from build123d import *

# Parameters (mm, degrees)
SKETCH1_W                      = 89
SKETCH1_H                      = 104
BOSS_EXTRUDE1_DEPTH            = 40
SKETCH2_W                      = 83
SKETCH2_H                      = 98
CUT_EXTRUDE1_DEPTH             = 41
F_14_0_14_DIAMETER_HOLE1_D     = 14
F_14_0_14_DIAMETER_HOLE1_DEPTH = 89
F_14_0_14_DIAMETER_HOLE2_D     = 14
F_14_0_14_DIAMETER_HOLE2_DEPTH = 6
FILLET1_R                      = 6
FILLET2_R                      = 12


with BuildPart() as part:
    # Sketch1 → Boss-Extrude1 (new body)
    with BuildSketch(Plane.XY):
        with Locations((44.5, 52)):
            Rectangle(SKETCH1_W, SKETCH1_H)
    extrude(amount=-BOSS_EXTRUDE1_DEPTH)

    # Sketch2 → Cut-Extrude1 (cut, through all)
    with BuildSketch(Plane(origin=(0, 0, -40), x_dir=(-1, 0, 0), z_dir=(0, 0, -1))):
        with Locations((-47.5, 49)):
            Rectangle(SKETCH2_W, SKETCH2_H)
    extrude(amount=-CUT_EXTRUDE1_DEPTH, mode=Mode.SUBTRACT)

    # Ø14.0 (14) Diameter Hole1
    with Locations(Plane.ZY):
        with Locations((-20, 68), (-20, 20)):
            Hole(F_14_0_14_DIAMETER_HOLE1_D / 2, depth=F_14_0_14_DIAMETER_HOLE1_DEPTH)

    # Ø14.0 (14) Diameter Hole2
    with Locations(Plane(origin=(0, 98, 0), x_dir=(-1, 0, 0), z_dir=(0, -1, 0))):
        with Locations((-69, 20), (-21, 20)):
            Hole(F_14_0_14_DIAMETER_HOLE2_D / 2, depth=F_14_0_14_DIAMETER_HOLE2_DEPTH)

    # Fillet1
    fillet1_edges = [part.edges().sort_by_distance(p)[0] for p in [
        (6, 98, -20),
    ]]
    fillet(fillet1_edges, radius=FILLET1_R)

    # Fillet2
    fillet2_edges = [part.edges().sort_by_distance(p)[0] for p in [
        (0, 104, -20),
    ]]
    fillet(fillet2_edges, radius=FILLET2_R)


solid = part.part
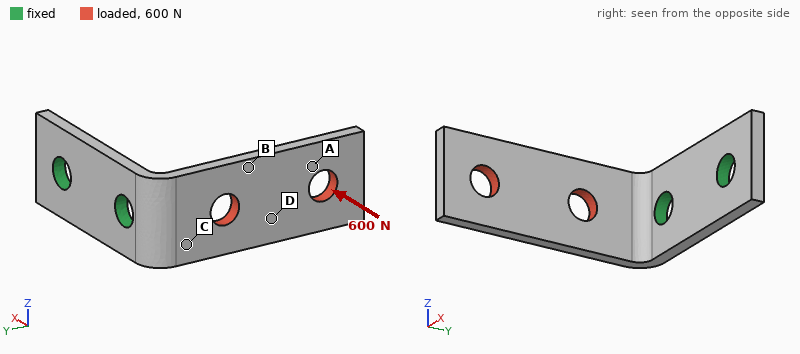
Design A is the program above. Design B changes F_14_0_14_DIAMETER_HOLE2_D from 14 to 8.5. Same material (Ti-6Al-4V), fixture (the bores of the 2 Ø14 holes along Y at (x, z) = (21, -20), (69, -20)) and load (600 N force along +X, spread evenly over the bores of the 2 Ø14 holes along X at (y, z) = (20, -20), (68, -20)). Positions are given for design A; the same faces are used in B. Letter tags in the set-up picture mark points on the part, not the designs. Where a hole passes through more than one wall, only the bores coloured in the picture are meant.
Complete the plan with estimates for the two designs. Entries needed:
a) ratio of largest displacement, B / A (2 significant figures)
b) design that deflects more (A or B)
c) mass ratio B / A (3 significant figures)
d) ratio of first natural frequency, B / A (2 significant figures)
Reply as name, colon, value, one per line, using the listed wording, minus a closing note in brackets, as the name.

ratio of largest displacement, B / A: 1.1
design that deflects more: B
mass ratio B / A: 1.03
ratio of first natural frequency, B / A: 0.96
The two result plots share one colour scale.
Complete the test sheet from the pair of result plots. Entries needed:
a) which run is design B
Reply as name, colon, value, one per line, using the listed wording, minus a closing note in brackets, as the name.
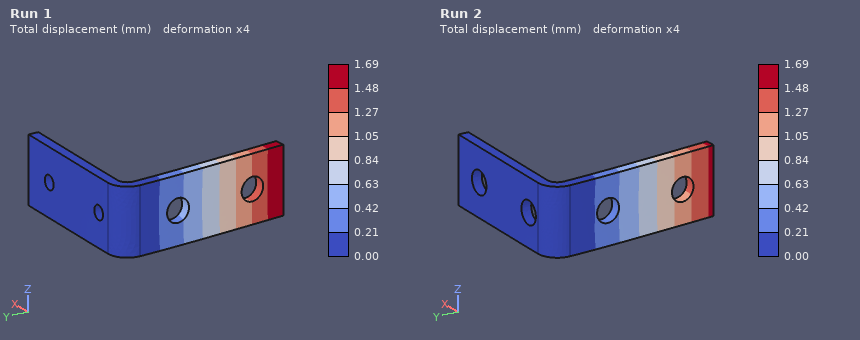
which run is design B: Run 1
